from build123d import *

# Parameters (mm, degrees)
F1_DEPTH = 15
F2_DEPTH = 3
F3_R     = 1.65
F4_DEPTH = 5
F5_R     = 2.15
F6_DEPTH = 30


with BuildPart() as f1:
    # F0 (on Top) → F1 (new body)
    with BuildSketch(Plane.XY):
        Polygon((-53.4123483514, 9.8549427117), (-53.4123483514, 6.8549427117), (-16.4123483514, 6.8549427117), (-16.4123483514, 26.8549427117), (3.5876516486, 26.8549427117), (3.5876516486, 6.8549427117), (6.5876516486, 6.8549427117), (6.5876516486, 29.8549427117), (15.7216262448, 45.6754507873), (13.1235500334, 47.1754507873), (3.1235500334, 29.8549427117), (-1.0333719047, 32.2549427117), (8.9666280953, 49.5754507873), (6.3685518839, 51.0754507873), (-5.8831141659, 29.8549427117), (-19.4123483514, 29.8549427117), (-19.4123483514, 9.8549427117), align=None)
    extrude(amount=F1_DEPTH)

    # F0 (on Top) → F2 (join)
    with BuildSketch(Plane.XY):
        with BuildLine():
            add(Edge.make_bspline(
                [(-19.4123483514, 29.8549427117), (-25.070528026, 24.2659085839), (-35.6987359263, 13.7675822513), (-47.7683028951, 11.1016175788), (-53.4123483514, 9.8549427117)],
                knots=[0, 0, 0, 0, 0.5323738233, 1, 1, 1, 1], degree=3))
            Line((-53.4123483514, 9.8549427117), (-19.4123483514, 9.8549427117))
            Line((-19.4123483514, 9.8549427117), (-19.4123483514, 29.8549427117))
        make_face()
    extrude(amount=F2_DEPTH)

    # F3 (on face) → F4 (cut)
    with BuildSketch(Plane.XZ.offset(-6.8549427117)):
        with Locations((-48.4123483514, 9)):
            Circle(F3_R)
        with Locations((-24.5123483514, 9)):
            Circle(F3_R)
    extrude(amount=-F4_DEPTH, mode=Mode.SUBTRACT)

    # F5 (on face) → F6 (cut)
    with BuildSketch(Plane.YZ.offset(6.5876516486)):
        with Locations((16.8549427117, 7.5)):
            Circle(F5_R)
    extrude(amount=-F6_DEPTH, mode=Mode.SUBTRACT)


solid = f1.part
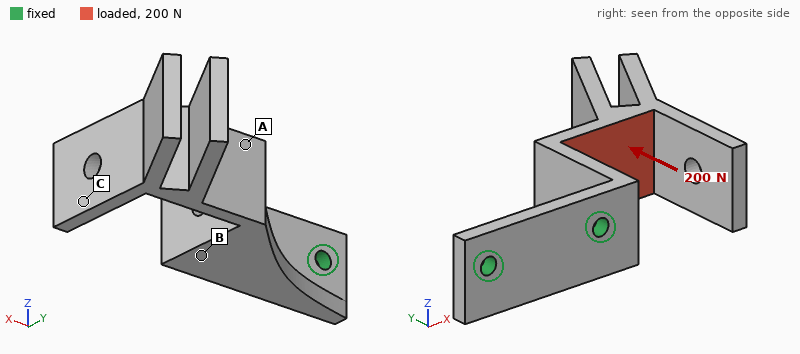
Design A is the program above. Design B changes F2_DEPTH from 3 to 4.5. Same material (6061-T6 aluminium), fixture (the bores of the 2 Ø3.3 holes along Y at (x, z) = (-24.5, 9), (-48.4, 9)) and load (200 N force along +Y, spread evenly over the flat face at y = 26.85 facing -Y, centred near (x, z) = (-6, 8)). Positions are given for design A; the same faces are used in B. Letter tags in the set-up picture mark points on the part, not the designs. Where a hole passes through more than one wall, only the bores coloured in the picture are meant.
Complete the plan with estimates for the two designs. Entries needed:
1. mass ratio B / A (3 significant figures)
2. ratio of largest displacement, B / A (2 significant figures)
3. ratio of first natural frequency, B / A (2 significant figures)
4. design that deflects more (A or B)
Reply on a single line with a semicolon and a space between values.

1.05; 0.86; 1.1; A
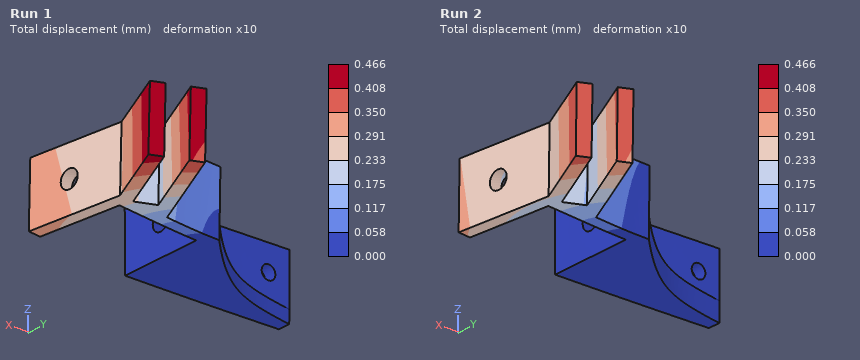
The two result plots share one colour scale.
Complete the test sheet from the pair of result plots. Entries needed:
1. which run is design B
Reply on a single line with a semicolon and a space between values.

Run 2
